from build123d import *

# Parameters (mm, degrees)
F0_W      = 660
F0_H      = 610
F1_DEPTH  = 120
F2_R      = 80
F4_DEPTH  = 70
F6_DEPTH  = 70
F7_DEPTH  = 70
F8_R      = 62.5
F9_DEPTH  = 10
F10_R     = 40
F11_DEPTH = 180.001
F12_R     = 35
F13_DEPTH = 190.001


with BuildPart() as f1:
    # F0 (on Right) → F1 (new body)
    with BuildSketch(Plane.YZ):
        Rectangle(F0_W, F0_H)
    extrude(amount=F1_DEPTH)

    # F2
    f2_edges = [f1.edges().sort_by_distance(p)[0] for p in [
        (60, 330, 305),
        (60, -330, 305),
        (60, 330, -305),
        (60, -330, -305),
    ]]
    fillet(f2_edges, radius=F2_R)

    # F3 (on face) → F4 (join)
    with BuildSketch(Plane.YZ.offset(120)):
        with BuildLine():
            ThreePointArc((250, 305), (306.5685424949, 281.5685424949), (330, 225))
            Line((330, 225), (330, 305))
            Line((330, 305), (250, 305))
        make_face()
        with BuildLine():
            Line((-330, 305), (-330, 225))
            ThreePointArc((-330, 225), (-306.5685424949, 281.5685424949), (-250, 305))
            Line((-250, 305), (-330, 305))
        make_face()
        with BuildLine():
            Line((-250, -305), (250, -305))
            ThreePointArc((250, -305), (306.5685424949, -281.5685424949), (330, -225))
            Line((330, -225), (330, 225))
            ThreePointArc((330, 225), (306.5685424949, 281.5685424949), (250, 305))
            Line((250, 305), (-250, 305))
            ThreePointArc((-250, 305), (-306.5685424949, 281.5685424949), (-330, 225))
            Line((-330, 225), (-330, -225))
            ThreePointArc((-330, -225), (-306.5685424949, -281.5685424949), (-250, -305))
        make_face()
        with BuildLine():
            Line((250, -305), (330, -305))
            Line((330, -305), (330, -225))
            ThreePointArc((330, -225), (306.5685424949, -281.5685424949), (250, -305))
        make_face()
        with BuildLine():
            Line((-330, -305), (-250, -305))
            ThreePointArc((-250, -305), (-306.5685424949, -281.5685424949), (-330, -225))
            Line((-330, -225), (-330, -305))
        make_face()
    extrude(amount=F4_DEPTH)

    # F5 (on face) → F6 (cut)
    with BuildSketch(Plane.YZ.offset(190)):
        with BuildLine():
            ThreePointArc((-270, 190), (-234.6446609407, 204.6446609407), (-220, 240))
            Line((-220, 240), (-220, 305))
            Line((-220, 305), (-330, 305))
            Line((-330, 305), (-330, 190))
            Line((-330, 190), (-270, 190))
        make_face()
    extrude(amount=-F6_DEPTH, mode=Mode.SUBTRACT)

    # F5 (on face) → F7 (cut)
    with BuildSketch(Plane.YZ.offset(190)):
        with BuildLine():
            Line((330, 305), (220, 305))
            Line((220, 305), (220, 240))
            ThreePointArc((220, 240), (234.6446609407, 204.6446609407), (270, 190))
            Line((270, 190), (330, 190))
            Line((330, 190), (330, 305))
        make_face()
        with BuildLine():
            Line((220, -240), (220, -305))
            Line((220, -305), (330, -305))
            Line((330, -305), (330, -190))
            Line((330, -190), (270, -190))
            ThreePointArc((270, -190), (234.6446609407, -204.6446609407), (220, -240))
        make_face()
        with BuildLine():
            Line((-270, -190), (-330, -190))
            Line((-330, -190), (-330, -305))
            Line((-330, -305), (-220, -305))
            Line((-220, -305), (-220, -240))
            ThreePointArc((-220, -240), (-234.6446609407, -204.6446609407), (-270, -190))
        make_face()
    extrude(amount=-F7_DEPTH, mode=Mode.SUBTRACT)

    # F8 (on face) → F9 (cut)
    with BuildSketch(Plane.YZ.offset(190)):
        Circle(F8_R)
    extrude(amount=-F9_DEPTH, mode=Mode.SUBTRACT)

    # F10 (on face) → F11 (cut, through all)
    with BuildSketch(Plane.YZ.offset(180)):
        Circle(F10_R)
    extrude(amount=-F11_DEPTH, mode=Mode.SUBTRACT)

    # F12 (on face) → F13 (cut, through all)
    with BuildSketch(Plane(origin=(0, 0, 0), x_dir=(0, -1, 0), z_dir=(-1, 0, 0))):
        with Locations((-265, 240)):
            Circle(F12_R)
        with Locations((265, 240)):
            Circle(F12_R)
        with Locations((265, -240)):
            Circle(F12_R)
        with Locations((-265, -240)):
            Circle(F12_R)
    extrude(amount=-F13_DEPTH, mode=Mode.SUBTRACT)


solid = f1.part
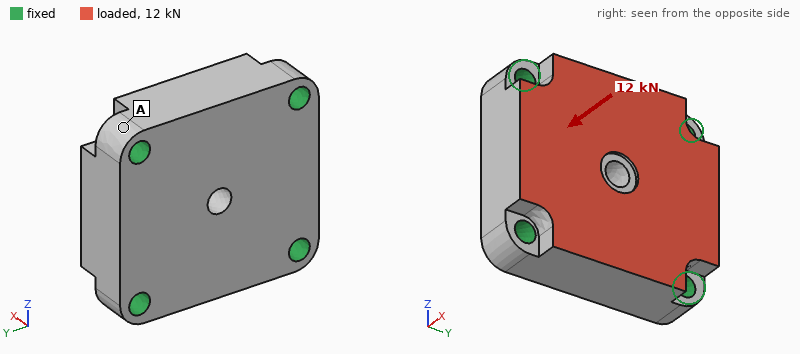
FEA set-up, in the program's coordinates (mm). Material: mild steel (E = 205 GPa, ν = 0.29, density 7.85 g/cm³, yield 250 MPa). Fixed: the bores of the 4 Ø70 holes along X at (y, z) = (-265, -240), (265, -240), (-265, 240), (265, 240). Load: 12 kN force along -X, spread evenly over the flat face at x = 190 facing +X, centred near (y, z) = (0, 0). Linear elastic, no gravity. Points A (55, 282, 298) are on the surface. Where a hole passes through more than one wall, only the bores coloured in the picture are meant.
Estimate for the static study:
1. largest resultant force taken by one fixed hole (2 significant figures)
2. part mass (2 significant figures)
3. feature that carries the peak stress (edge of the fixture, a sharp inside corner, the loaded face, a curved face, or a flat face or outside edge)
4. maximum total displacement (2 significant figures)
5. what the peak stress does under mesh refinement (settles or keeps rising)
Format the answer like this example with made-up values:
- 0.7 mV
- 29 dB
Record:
- 3.2 kN
- 550 kg
- edge of the fixture
- 0.32 µm
- keeps rising
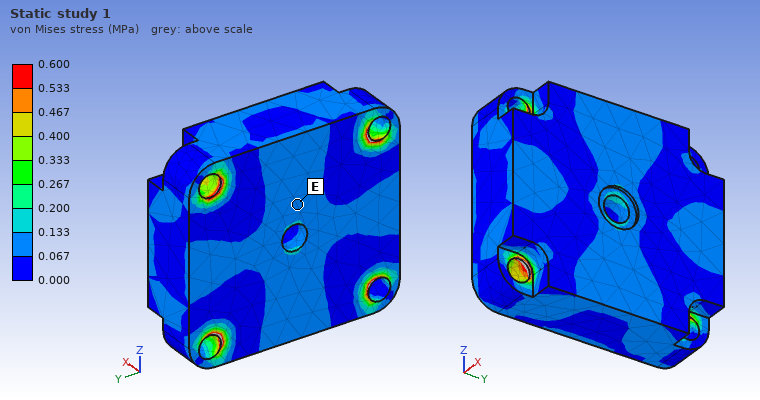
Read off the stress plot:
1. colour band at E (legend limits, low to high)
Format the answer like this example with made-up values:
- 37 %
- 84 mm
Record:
- 0.067 to 0.133 MPa
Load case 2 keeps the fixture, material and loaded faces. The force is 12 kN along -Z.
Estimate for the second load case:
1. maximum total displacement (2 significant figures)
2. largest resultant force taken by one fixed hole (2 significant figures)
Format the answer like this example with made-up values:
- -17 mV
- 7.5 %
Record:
- 0.31 µm
- 3.5 kN
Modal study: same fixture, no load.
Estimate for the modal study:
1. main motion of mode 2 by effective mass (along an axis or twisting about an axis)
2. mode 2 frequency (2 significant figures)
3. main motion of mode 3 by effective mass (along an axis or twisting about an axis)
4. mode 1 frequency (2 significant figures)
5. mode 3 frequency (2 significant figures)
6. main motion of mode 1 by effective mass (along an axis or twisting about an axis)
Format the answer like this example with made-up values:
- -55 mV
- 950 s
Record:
- twisting about Y
- 2200 Hz
- along Z
- 1500 Hz
- 2300 Hz
- along X
